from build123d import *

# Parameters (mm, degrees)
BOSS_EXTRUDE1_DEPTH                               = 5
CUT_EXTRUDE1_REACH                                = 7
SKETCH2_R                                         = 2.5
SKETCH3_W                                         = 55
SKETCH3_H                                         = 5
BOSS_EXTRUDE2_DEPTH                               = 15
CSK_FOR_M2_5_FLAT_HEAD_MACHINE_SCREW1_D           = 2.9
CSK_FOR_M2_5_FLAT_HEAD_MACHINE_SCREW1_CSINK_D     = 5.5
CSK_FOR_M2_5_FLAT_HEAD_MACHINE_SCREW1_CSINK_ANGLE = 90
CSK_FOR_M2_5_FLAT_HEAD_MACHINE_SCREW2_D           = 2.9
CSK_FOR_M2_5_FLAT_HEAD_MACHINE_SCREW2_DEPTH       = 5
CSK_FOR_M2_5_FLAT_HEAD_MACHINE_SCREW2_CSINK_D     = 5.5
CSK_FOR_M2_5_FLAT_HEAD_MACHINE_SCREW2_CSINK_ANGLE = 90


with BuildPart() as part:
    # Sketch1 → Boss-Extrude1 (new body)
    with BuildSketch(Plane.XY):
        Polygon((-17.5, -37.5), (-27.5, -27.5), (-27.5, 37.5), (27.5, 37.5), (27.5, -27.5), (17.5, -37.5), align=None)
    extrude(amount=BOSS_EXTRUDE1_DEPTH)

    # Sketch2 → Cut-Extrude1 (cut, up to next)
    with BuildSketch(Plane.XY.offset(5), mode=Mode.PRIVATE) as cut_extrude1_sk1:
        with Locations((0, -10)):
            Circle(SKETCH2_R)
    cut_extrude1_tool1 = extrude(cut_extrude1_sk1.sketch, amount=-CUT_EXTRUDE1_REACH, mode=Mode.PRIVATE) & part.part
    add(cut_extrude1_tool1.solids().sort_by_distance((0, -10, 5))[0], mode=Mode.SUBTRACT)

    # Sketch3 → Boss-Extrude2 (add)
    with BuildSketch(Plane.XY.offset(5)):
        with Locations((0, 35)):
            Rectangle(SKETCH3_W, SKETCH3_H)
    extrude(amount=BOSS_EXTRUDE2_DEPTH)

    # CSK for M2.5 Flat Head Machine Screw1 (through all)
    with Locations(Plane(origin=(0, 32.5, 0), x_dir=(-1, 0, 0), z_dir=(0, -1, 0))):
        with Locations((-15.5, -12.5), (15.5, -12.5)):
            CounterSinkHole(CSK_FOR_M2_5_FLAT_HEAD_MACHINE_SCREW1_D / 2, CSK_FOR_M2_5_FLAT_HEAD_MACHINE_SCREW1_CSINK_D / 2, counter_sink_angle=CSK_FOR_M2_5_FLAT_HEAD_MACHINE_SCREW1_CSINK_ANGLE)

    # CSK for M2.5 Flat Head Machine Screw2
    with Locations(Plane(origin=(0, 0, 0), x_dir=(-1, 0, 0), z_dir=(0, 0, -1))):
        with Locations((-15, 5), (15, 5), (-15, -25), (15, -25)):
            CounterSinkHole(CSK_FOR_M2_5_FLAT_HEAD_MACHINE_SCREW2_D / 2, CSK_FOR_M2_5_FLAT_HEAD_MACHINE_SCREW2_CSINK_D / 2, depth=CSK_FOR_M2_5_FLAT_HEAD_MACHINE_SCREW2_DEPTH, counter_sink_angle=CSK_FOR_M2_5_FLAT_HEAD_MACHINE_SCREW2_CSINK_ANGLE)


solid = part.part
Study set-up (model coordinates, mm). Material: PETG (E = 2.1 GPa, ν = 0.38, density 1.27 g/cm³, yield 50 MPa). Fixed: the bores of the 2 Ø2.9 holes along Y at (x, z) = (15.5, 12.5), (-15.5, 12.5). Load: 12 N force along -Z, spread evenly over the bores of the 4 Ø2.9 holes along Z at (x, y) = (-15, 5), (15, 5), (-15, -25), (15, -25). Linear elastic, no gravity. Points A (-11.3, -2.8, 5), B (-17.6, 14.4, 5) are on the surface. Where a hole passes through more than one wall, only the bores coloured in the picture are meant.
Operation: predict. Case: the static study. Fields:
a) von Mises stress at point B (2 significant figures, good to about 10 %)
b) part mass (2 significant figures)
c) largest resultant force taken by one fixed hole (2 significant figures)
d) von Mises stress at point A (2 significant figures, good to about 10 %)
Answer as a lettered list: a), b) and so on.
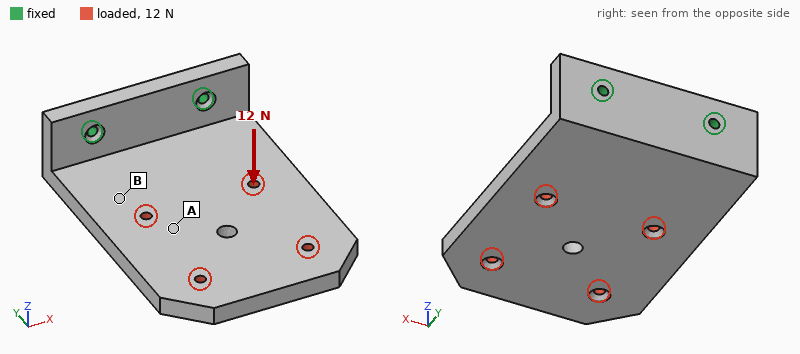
a) 1.2 MPa
b) 30 g
c) 7.1 N
d) 0.59 MPa
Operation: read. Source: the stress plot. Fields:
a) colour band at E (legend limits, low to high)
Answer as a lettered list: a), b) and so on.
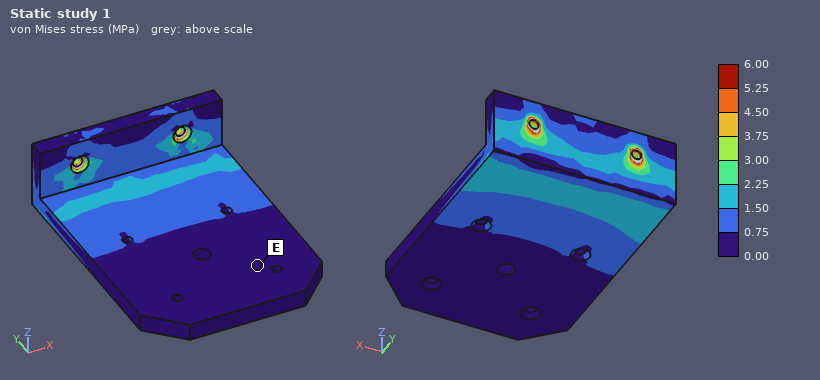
a) 0.00 to 0.75 MPa
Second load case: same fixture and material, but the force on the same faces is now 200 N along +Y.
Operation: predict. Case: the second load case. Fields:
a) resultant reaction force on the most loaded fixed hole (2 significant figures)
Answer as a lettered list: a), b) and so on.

a) 100 N
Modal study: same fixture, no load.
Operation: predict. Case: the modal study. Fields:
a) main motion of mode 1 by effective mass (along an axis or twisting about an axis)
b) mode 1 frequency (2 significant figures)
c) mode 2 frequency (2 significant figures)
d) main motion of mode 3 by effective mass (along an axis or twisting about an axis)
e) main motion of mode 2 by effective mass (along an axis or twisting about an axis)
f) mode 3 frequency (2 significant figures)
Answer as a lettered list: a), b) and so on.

a) along Z
b) 160 Hz
c) 490 Hz
d) along X
e) along X
f) 680 Hz
